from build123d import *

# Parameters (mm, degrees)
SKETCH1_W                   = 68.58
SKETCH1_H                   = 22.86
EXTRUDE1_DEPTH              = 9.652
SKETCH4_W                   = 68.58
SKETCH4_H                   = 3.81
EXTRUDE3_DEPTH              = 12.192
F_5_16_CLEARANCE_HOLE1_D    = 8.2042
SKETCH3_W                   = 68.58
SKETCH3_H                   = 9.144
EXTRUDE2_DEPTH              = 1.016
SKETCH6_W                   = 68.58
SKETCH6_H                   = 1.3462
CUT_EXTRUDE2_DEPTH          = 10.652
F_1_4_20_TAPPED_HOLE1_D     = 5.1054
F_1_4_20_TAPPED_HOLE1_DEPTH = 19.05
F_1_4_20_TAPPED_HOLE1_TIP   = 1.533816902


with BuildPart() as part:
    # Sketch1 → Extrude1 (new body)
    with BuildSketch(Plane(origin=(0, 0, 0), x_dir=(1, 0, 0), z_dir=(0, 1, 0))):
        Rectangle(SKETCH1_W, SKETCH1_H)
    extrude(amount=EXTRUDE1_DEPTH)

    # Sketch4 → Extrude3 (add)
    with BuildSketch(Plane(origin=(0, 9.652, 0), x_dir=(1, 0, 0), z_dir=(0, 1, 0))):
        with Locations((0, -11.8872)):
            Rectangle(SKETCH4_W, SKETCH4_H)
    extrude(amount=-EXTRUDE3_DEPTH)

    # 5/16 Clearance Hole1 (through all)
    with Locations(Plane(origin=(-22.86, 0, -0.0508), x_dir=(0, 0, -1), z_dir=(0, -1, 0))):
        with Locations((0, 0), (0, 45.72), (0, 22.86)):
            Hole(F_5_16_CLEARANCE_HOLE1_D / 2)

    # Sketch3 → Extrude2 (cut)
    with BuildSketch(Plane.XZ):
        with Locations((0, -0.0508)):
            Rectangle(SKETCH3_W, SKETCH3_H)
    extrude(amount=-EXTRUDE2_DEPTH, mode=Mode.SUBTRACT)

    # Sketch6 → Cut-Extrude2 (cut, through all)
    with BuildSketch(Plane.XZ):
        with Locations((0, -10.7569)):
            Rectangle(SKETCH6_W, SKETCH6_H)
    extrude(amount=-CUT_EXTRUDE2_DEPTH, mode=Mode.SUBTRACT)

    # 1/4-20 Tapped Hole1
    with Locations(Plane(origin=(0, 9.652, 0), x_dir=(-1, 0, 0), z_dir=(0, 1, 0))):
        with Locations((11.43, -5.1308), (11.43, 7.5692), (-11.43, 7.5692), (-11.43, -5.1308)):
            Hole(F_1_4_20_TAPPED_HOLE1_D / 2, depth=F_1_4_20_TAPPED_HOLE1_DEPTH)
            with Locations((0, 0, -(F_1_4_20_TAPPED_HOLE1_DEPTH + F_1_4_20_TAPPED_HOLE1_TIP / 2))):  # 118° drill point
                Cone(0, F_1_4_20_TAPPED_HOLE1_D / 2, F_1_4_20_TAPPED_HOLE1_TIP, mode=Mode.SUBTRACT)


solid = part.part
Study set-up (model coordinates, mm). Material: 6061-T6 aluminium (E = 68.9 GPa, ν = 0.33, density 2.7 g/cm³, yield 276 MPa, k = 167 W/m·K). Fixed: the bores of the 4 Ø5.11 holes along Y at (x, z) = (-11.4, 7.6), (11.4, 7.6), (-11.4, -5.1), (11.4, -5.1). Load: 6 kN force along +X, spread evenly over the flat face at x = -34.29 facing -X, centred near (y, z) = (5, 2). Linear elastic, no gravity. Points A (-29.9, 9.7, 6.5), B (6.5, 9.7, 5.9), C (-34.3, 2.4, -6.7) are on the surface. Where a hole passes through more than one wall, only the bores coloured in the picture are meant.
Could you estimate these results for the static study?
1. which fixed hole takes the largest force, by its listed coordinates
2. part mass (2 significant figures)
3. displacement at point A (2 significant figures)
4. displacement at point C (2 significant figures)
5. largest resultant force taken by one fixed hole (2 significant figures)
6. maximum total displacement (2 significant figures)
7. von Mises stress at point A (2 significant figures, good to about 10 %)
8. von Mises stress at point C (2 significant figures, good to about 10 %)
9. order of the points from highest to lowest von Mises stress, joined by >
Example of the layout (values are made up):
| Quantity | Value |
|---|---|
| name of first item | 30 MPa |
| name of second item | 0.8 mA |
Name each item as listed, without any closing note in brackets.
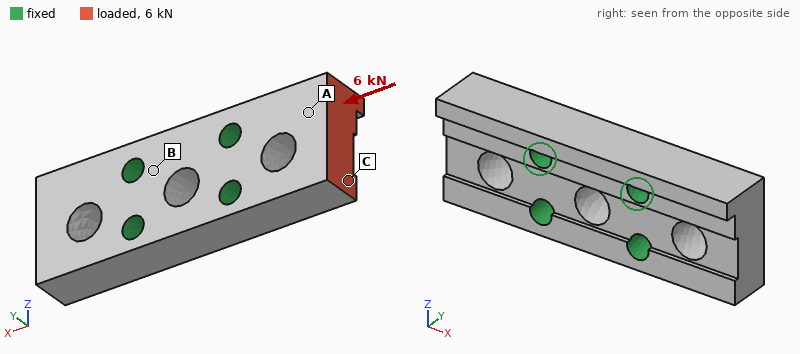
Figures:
| Quantity | Value |
|---|---|
| which fixed hole takes the largest force, by its listed coordinates | (-11.4, 7.6) |
| part mass | 37 g |
| displacement at point A | 9.5 µm |
| displacement at point C | 11 µm |
| largest resultant force taken by one fixed hole | 3.3 kN |
| maximum total displacement | 14 µm |
| von Mises stress at point A | 36 MPa |
| von Mises stress at point C | 25 MPa |
| order of the points from highest to lowest von Mises stress, joined by > | A > C > B |
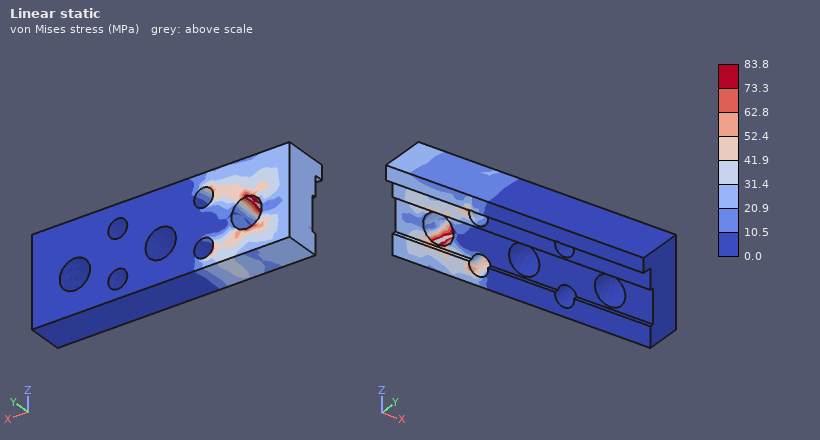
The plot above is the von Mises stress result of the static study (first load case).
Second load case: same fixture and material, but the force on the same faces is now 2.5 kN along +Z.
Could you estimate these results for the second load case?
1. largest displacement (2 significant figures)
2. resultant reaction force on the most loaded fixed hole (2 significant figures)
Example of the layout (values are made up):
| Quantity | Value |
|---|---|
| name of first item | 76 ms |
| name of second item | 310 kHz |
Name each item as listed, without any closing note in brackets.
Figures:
| Quantity | Value |
|---|---|
| largest displacement | 43 µm |
| resultant reaction force on the most loaded fixed hole | 3.2 kN |
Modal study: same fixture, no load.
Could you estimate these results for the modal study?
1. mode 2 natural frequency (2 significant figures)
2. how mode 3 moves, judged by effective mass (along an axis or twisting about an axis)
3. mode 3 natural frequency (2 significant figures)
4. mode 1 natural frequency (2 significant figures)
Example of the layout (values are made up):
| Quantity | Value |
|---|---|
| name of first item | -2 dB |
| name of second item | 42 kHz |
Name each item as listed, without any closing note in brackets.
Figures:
| Quantity | Value |
|---|---|
| mode 2 natural frequency | 14 kHz |
| how mode 3 moves, judged by effective mass | twisting about Y |
| mode 3 natural frequency | 20 kHz |
| mode 1 natural frequency | 14 kHz |
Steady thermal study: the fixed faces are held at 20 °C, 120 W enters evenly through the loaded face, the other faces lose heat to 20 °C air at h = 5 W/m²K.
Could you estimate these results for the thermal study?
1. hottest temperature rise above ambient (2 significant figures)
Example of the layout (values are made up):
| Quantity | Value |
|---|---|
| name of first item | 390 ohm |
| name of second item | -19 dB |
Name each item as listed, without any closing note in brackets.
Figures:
| Quantity | Value |
|---|---|
| hottest temperature rise above ambient | 82 K |
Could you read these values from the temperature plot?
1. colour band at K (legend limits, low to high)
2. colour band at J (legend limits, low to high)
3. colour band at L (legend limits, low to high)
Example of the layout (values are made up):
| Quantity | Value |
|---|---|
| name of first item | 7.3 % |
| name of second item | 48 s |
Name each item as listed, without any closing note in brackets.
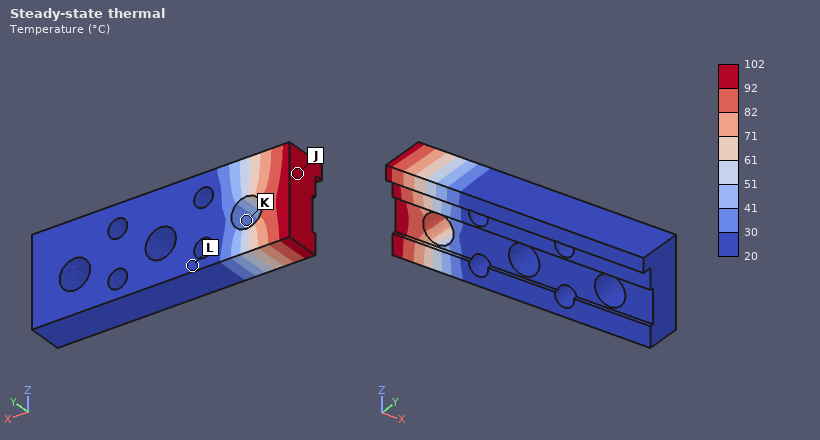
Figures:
| Quantity | Value |
|---|---|
| colour band at K | 30 to 41 °C |
| colour band at J | 92 to 102 °C |
| colour band at L | 20 to 30 °C |
